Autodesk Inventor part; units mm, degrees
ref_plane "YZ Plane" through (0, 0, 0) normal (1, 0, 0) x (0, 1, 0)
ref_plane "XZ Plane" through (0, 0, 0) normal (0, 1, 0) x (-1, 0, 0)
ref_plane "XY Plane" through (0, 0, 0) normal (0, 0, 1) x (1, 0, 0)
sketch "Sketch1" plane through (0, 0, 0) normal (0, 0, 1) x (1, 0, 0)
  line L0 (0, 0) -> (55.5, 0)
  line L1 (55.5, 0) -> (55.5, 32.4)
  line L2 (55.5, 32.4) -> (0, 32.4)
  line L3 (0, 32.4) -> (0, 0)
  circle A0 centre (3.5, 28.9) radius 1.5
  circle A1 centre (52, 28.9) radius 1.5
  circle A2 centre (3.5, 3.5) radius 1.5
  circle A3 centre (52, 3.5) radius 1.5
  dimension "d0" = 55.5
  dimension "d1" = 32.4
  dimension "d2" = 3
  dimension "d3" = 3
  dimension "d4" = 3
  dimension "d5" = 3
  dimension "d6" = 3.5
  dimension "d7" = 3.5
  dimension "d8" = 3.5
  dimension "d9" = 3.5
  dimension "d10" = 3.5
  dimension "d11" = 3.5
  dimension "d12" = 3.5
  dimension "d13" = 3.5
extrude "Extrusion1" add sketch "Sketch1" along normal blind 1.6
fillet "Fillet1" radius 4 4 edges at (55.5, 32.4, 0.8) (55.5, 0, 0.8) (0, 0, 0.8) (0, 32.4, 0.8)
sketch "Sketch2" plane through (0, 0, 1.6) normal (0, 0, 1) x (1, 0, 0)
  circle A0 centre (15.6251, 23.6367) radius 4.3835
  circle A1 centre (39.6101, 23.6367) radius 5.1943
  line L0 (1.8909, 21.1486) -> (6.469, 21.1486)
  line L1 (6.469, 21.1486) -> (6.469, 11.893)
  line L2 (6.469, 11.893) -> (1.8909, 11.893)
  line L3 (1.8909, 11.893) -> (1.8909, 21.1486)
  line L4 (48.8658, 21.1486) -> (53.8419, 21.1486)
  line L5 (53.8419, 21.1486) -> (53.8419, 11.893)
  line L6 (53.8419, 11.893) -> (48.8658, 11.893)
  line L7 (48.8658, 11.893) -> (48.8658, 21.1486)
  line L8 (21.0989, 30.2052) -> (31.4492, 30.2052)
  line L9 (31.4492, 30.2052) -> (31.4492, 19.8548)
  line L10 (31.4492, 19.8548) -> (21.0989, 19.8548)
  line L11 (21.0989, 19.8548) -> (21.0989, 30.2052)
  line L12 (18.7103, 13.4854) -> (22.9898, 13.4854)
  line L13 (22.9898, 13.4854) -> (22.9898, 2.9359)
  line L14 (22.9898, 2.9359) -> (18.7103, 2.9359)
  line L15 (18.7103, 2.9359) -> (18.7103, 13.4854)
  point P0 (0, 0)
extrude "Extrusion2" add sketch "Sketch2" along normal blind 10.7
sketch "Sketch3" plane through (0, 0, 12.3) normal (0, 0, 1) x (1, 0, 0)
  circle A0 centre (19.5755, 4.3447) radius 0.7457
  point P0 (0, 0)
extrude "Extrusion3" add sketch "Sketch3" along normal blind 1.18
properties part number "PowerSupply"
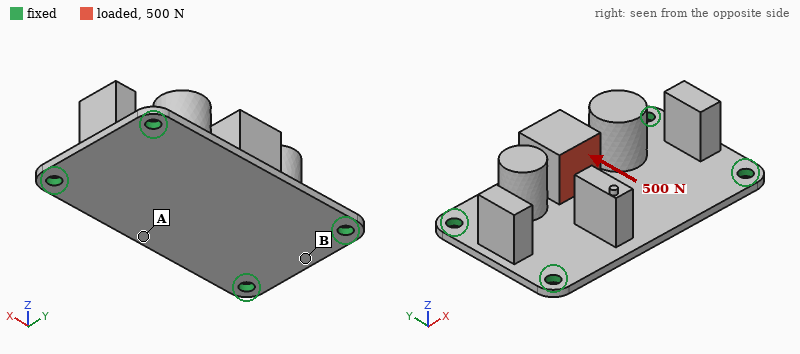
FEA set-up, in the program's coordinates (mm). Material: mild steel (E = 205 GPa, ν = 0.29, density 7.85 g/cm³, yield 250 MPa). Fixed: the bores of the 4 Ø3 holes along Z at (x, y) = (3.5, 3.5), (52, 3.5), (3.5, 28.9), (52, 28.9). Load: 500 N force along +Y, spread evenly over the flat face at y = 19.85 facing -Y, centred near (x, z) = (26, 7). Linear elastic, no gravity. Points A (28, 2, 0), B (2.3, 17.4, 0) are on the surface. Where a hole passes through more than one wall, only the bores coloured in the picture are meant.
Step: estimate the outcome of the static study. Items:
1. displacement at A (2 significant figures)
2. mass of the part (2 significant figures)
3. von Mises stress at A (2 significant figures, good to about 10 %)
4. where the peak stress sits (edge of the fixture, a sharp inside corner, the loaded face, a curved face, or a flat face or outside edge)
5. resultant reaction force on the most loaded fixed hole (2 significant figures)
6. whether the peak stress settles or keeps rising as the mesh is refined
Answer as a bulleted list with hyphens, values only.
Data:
- 24 µm
- 54 g
- 32 MPa
- edge of the fixture
- 200 N
- keeps rising
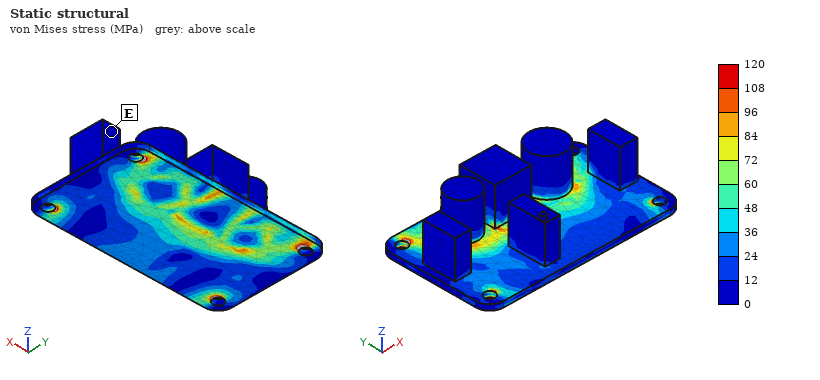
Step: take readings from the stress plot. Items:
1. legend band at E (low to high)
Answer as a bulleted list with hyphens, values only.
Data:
- 0 to 12 MPa
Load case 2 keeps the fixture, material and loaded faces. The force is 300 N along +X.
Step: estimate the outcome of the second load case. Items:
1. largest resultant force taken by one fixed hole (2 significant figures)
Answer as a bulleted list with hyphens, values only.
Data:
- 120 N
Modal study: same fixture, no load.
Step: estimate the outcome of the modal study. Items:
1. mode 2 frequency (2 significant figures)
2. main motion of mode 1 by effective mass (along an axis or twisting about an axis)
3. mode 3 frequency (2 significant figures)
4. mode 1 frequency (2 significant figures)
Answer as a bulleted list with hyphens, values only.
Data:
- 3500 Hz
- along Z
- 5200 Hz
- 2200 Hz
